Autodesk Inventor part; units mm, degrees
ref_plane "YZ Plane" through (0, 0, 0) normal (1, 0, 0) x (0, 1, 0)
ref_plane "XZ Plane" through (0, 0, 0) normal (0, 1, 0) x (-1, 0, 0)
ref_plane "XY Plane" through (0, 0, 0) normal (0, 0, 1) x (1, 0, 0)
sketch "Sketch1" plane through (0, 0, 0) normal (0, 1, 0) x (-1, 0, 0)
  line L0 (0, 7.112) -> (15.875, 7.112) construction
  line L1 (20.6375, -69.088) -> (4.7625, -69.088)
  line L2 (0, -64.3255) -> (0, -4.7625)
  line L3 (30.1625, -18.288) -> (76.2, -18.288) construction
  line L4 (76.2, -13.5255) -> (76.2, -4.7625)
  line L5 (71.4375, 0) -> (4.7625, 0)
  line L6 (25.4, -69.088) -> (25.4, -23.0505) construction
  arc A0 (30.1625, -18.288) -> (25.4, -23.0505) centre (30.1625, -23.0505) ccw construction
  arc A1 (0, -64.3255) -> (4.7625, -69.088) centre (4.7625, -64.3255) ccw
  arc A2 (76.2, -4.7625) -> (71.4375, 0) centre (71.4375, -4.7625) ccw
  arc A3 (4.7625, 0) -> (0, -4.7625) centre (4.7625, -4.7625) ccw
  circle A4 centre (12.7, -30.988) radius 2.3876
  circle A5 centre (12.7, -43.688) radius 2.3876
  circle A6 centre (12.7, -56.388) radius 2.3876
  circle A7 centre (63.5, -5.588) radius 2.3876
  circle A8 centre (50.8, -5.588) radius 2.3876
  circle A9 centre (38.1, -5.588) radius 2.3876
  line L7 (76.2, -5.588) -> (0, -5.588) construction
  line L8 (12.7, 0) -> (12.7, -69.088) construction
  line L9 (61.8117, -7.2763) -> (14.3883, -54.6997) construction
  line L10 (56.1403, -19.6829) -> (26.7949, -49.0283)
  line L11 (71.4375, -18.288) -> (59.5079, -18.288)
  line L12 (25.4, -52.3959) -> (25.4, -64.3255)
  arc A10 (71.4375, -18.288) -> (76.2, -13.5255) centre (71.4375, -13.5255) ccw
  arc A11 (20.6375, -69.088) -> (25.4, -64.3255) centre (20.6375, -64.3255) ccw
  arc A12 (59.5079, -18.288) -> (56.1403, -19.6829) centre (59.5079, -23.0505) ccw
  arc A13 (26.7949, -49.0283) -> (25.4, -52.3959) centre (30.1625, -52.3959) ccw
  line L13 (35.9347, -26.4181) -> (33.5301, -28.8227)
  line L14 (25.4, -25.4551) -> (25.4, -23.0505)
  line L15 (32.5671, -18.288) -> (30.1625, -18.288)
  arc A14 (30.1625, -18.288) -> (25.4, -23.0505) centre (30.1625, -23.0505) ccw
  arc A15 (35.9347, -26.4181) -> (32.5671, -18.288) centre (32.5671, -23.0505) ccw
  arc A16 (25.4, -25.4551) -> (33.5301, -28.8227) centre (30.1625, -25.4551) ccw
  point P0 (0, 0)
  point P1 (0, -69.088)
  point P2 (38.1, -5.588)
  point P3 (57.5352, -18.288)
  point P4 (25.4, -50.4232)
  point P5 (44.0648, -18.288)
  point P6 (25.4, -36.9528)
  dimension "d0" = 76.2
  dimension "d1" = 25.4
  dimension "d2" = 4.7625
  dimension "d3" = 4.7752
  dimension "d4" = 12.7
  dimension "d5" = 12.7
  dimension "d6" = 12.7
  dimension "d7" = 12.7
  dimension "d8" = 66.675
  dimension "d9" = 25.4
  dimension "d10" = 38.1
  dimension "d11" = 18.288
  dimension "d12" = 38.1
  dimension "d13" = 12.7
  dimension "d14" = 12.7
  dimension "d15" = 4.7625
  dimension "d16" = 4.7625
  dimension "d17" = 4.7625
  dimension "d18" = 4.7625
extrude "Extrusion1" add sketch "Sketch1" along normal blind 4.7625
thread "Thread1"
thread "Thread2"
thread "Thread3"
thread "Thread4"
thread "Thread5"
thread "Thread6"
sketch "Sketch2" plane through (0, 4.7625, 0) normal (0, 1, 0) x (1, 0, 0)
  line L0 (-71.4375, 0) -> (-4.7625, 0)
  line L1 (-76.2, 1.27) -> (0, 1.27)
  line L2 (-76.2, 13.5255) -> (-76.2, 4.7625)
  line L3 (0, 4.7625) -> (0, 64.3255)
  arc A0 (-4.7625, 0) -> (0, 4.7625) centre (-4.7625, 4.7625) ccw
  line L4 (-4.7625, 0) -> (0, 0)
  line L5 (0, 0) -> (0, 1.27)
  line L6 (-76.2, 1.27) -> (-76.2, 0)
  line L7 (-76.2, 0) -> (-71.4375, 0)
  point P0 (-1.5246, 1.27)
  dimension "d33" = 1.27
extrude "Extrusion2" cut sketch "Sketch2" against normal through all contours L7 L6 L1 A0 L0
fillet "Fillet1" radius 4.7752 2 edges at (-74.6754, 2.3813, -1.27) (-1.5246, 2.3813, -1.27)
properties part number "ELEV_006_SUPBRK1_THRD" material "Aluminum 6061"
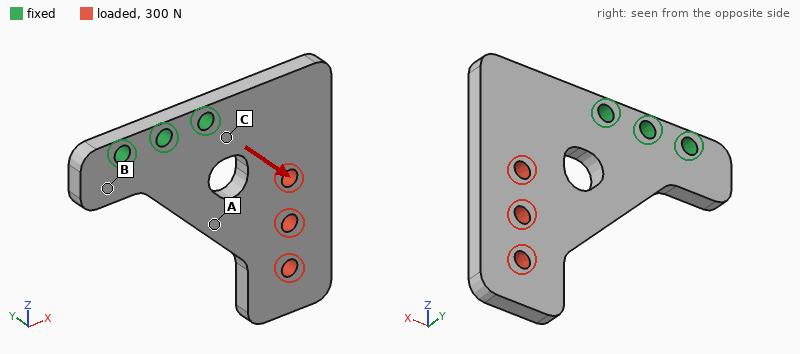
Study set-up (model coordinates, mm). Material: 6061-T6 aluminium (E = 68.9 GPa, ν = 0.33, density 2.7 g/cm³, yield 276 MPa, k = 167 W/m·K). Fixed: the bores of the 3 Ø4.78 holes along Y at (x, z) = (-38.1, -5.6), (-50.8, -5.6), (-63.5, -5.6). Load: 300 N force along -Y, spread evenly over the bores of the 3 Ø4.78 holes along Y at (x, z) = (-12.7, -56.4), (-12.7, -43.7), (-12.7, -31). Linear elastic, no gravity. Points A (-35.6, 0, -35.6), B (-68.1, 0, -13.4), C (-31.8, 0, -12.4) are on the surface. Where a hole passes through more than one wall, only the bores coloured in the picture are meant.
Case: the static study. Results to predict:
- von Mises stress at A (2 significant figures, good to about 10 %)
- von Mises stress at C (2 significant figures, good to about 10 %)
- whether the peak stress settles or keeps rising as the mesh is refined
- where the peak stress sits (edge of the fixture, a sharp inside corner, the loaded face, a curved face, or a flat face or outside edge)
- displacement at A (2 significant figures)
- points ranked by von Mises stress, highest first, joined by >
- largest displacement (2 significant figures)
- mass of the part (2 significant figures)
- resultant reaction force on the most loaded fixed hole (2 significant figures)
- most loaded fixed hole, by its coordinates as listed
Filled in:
60 MPa
89 MPa
keeps rising
edge of the fixture
0.20 mm
C > A > B
0.98 mm
37 g
530 N
(-38.1, -5.6)
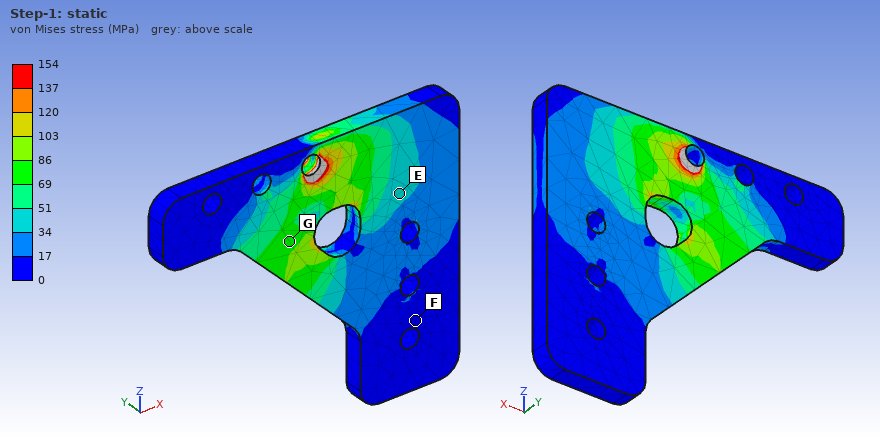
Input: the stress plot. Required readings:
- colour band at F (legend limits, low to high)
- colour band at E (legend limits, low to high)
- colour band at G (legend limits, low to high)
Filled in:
0 to 17 MPa
34 to 51 MPa
69 to 86 MPa
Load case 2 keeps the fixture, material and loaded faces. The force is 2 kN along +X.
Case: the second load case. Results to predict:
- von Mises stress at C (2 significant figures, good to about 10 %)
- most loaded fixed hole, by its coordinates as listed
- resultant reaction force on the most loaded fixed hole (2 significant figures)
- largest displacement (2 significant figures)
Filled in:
31 MPa
(-38.1, -5.6)
3.1 kN
0.20 mm
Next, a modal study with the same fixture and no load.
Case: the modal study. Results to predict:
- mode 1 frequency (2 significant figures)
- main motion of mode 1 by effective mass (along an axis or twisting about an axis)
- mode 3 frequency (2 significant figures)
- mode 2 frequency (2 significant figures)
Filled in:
860 Hz
along Y
3800 Hz
2400 Hz
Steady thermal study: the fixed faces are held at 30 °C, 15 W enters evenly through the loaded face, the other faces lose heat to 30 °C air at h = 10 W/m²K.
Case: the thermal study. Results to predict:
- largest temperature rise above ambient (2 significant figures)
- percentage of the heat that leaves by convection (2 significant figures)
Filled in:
29 K
6.9 %
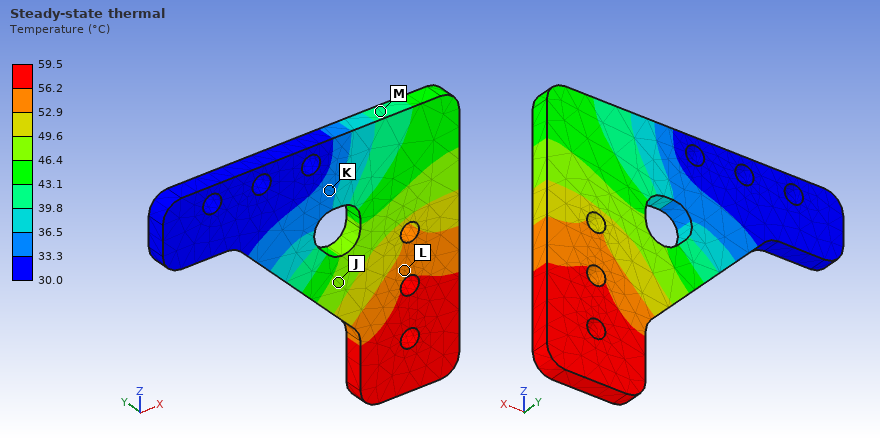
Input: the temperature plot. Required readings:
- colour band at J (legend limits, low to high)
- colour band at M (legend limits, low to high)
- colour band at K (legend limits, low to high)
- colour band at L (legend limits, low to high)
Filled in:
46.4 to 49.6 °C
39.8 to 43.1 °C
33.3 to 36.5 °C
52.9 to 56.2 °C
